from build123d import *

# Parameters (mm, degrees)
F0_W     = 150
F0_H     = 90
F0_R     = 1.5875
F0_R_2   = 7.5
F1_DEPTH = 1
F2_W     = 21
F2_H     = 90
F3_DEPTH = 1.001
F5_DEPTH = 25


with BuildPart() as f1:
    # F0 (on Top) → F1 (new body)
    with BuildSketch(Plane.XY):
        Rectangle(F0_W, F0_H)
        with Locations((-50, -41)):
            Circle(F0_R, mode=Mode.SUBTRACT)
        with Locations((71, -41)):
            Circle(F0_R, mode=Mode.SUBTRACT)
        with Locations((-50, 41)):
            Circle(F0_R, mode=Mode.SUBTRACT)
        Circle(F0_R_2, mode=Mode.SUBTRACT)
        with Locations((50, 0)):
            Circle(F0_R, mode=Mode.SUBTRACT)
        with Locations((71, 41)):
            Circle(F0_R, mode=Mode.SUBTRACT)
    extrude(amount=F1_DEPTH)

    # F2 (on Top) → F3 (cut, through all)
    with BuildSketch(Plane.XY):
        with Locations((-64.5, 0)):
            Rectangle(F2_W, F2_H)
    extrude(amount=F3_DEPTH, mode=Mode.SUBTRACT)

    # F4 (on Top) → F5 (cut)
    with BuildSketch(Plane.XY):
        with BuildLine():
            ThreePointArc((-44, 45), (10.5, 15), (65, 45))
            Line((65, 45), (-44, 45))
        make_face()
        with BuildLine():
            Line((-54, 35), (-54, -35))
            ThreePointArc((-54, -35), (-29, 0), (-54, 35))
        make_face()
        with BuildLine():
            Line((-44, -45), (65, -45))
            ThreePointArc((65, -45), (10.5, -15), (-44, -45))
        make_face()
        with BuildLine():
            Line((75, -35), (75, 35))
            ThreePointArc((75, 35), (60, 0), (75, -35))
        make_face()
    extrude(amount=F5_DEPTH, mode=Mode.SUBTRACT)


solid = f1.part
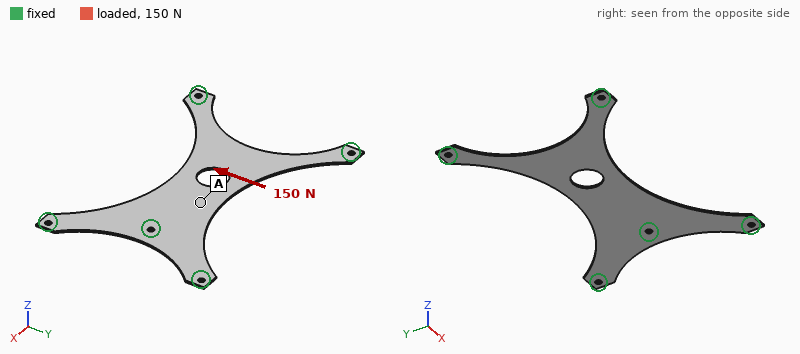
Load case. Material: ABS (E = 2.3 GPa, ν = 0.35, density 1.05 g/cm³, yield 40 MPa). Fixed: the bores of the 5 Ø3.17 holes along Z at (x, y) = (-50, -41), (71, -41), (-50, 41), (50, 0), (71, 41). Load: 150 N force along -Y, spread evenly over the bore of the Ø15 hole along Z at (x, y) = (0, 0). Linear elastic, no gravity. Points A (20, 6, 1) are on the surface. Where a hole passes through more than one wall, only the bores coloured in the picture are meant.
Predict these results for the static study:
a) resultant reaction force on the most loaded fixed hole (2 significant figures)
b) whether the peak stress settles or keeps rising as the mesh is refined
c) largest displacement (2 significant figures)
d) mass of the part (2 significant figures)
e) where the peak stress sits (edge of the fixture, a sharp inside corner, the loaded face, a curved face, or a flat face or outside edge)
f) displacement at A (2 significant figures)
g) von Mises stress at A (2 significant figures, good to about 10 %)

65 N
keeps rising
0.25 mm
5.0 g
edge of the fixture
0.16 mm
3.6 MPa
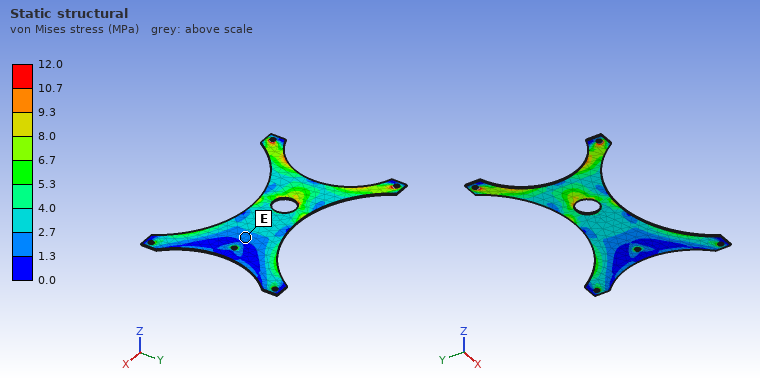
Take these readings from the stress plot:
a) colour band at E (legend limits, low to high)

1.3 to 2.7 MPa
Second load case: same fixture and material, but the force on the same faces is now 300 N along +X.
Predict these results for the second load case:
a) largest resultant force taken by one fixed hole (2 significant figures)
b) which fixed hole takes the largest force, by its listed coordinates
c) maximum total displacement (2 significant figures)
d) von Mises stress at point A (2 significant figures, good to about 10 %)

160 N
(50, 0)
0.20 mm
6.3 MPa
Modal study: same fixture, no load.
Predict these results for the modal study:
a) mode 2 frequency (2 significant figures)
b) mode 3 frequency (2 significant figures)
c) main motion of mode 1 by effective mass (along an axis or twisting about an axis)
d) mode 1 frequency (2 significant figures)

290 Hz
300 Hz
along Z
120 Hz
